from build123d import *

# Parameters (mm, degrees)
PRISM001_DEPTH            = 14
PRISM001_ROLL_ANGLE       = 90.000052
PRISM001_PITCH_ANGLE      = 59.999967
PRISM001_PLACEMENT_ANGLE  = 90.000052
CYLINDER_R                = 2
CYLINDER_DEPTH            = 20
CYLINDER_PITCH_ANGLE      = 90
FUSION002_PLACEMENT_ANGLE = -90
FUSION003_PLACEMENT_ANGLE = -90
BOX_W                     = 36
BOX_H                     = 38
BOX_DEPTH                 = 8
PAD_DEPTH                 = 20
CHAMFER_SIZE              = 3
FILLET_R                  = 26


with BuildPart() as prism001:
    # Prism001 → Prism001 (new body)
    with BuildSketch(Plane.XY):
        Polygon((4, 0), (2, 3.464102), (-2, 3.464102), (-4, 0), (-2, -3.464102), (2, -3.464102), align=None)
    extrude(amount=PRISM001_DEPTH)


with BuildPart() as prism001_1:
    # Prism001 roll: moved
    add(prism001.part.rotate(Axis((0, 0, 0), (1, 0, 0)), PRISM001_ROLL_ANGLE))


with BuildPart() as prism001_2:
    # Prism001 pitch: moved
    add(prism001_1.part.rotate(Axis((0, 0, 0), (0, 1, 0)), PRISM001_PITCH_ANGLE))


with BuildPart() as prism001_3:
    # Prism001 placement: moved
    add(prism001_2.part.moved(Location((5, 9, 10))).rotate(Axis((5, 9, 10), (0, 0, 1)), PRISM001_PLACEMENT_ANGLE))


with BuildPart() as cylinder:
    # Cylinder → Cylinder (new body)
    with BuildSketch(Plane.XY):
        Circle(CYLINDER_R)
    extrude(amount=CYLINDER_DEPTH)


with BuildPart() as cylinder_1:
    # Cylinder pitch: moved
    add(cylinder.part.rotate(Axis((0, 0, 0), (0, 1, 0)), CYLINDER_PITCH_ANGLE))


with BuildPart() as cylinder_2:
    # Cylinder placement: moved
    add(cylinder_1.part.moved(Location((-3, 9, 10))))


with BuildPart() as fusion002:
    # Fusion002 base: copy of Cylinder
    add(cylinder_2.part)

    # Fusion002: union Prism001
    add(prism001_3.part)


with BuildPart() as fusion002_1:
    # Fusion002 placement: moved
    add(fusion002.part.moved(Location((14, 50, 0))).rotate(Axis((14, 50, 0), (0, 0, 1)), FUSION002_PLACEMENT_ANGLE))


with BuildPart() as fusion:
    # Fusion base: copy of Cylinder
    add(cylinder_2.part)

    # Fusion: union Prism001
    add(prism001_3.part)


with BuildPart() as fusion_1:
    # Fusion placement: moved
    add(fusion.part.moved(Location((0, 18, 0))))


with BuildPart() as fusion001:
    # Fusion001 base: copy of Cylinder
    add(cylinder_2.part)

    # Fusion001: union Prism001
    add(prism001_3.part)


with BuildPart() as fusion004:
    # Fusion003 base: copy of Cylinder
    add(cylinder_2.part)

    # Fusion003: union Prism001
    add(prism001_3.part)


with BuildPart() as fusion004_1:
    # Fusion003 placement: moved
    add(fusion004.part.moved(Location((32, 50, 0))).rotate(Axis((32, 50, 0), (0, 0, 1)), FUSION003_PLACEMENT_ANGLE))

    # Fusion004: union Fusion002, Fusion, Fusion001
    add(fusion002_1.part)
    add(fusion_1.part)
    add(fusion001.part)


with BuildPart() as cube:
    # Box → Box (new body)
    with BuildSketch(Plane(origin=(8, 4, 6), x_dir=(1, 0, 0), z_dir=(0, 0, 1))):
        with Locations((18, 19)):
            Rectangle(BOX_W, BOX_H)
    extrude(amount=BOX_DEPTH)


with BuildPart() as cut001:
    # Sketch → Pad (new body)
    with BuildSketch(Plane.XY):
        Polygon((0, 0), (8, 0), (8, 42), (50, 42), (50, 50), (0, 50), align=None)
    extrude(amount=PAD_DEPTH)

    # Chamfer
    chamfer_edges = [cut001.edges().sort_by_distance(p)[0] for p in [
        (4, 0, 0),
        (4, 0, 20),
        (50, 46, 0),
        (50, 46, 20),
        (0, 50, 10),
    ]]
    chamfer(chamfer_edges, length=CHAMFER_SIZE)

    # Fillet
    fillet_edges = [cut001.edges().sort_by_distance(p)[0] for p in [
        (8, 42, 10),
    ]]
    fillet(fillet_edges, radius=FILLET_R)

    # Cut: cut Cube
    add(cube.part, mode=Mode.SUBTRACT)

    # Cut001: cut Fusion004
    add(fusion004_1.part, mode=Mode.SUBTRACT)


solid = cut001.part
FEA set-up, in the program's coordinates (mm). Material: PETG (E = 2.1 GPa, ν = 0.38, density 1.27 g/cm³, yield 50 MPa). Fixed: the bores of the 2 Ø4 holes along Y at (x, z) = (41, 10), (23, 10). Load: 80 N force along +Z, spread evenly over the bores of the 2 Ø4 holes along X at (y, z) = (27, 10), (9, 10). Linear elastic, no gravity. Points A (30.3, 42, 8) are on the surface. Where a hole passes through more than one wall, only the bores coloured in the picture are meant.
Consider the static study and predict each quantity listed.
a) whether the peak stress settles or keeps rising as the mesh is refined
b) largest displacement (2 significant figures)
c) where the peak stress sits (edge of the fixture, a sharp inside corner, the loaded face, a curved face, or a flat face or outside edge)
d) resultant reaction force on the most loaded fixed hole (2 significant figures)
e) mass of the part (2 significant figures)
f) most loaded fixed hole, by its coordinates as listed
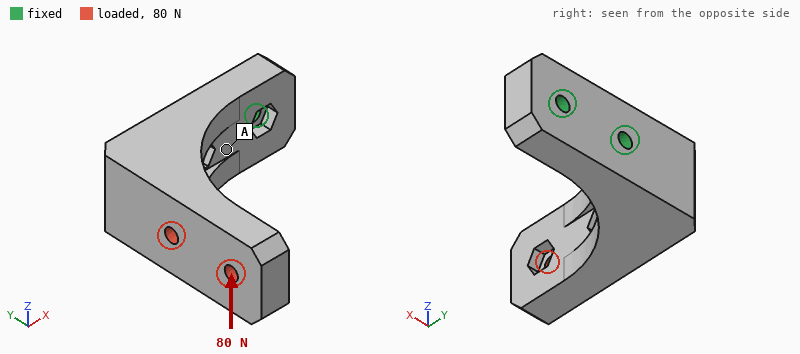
keeps rising
0.83 mm
edge of the fixture
140 N
20 g
(23, 10)
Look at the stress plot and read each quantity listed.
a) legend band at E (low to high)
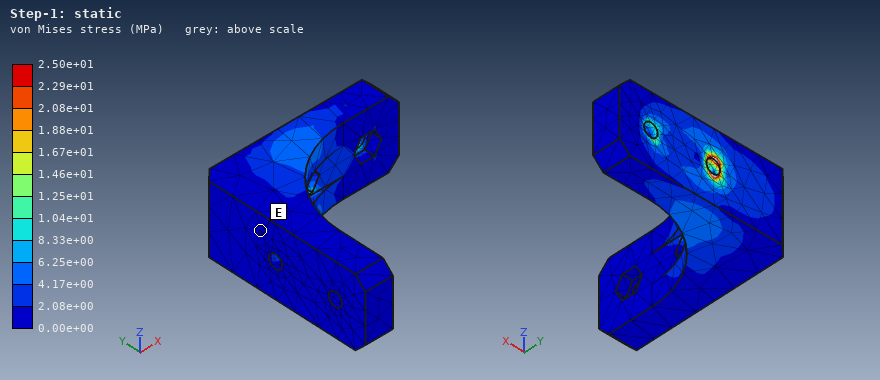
0.00e+00 to 2.08e+00 MPa
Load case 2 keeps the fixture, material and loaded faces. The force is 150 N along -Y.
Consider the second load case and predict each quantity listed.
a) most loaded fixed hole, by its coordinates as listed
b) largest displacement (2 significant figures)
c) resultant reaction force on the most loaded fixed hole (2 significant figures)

(23, 10)
0.67 mm
280 N
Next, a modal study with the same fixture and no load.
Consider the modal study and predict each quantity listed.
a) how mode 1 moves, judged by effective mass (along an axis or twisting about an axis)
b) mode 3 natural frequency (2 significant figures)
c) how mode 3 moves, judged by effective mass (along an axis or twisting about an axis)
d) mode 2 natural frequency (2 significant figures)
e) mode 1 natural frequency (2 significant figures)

along Z
2300 Hz
along Y
730 Hz
680 Hz
